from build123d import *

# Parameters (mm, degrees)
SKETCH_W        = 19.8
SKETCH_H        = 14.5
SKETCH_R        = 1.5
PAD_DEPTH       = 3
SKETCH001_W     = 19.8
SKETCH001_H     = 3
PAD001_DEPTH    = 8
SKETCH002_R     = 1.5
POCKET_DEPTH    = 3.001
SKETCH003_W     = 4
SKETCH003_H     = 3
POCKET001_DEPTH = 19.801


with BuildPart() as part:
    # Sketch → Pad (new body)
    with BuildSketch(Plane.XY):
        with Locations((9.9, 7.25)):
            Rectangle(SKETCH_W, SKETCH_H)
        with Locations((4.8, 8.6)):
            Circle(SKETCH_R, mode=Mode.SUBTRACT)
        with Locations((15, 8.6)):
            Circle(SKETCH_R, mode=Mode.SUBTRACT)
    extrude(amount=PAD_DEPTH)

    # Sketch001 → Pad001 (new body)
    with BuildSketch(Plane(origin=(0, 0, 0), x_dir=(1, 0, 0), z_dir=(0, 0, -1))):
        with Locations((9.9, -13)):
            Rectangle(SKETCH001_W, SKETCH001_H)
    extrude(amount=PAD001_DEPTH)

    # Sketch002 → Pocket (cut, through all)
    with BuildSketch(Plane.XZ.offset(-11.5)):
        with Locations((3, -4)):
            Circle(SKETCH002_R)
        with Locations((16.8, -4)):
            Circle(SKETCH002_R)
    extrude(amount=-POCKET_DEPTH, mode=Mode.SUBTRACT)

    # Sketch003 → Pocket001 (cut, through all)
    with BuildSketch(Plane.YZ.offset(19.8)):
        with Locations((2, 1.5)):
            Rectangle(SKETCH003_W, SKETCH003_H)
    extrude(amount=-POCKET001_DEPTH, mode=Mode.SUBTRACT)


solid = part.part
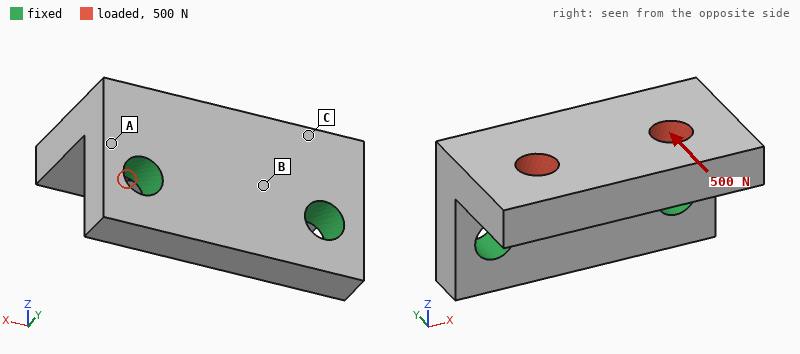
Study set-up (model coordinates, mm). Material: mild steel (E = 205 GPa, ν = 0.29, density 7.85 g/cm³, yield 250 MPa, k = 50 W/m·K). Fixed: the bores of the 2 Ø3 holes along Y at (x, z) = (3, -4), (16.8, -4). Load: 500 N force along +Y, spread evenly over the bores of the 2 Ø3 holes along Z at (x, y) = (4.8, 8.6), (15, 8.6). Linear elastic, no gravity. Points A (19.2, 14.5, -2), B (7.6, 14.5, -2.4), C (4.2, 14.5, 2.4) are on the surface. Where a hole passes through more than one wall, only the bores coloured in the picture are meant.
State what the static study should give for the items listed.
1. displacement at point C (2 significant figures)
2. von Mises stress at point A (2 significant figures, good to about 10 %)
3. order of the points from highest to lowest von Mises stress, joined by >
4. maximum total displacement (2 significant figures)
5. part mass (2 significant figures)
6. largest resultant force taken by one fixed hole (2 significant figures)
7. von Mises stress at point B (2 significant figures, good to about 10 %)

3.9 µm
57 MPa
A > B > C
8.3 µm
8.0 g
250 N
28 MPa
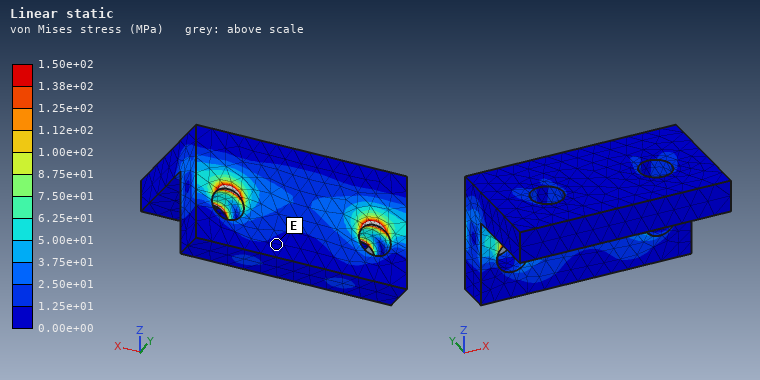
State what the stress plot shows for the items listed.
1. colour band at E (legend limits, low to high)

0.00e+00 to 1.25e+01 MPa
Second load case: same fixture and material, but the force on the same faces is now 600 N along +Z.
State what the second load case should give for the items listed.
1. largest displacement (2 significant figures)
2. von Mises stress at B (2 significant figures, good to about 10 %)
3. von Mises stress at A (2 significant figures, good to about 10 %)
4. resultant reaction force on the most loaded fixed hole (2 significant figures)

18 µm
46 MPa
76 MPa
310 N
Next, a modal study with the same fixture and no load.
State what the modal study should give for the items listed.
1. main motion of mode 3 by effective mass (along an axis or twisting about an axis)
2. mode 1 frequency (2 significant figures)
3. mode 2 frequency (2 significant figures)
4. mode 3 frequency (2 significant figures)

along X
16 kHz
27 kHz
40 kHz
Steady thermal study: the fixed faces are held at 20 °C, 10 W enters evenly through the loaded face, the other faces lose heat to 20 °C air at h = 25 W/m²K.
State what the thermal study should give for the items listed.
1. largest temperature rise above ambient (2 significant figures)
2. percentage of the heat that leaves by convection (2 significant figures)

35 K
3.6 %
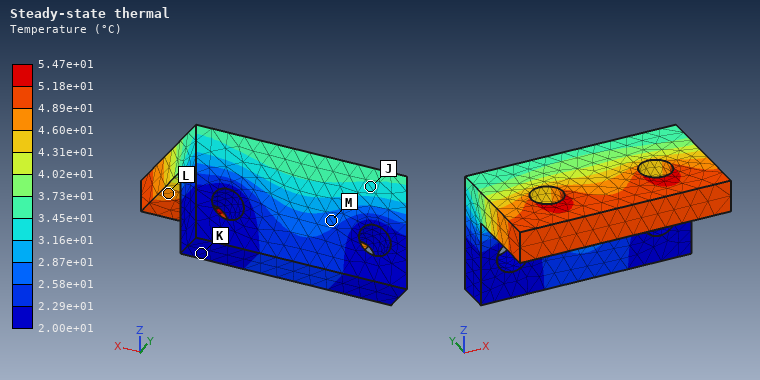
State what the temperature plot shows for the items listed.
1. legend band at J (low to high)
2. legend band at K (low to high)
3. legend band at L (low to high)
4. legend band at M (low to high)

3.16e+01 to 3.45e+01 °C
2.00e+01 to 2.29e+01 °C
4.60e+01 to 4.89e+01 °C
2.58e+01 to 2.87e+01 °C
